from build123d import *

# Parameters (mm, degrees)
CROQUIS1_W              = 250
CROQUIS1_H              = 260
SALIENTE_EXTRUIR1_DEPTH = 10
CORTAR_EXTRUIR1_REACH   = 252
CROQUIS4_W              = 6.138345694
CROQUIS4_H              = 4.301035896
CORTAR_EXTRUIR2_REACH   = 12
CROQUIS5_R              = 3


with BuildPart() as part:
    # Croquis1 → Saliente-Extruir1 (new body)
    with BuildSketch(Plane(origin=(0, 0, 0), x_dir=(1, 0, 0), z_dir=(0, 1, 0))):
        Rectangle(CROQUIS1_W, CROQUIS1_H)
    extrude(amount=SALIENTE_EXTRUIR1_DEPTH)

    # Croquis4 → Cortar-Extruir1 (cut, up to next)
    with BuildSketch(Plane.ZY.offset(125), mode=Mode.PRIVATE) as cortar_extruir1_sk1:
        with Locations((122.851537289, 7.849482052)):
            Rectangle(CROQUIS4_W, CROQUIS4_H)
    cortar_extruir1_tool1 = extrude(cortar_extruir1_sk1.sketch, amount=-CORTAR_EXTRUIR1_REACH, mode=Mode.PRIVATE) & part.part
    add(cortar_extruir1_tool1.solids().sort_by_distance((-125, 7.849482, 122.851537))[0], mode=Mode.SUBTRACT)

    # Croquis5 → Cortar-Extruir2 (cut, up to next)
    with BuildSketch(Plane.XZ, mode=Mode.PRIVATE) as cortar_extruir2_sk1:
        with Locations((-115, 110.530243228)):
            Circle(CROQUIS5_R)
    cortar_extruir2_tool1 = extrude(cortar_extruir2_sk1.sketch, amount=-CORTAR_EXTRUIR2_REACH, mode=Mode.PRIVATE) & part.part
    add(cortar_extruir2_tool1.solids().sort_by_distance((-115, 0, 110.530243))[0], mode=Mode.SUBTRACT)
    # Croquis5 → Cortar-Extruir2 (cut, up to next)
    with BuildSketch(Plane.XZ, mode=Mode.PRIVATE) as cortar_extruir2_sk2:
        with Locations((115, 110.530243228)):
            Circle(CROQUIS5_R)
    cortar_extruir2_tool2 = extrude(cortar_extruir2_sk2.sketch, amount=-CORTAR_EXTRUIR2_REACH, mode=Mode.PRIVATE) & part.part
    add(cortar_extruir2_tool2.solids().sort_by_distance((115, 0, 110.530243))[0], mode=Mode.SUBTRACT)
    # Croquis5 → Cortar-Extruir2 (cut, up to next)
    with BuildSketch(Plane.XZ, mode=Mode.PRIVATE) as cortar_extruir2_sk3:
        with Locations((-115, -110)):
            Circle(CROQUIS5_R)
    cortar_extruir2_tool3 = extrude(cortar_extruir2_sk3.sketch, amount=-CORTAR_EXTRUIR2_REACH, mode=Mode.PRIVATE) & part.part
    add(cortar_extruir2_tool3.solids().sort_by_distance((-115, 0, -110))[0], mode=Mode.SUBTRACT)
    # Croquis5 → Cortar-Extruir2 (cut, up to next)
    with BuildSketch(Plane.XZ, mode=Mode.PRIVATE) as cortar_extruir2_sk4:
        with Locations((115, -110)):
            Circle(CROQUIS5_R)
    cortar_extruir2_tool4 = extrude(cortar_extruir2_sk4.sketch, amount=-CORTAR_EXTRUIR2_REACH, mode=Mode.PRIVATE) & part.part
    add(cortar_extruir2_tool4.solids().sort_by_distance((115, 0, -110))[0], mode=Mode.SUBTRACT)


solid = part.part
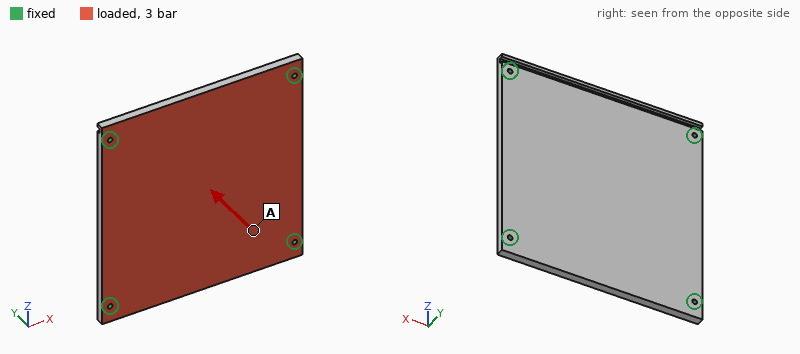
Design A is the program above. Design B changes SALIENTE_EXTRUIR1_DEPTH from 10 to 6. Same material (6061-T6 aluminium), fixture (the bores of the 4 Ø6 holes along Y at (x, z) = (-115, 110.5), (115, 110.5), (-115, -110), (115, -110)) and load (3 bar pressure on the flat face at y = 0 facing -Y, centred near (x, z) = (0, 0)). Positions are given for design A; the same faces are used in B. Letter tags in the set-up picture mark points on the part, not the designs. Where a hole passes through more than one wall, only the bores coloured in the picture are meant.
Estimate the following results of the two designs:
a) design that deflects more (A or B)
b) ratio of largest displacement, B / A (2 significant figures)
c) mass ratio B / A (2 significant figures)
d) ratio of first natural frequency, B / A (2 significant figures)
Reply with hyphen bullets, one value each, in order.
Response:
- B
- 4.3
- 0.61
- 0.63
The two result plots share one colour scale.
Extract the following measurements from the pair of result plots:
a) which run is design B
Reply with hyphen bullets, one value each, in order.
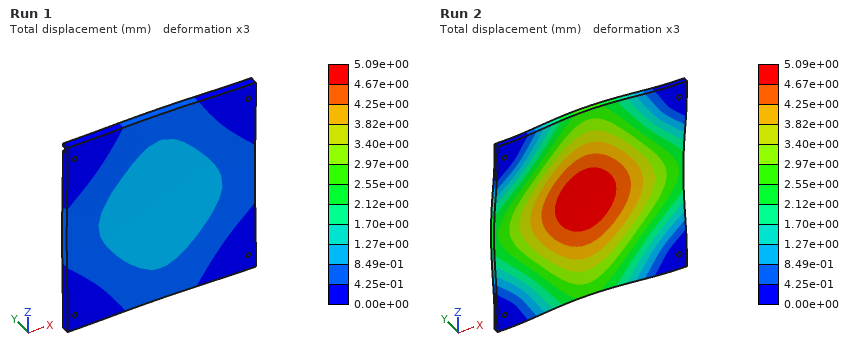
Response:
- Run 2
